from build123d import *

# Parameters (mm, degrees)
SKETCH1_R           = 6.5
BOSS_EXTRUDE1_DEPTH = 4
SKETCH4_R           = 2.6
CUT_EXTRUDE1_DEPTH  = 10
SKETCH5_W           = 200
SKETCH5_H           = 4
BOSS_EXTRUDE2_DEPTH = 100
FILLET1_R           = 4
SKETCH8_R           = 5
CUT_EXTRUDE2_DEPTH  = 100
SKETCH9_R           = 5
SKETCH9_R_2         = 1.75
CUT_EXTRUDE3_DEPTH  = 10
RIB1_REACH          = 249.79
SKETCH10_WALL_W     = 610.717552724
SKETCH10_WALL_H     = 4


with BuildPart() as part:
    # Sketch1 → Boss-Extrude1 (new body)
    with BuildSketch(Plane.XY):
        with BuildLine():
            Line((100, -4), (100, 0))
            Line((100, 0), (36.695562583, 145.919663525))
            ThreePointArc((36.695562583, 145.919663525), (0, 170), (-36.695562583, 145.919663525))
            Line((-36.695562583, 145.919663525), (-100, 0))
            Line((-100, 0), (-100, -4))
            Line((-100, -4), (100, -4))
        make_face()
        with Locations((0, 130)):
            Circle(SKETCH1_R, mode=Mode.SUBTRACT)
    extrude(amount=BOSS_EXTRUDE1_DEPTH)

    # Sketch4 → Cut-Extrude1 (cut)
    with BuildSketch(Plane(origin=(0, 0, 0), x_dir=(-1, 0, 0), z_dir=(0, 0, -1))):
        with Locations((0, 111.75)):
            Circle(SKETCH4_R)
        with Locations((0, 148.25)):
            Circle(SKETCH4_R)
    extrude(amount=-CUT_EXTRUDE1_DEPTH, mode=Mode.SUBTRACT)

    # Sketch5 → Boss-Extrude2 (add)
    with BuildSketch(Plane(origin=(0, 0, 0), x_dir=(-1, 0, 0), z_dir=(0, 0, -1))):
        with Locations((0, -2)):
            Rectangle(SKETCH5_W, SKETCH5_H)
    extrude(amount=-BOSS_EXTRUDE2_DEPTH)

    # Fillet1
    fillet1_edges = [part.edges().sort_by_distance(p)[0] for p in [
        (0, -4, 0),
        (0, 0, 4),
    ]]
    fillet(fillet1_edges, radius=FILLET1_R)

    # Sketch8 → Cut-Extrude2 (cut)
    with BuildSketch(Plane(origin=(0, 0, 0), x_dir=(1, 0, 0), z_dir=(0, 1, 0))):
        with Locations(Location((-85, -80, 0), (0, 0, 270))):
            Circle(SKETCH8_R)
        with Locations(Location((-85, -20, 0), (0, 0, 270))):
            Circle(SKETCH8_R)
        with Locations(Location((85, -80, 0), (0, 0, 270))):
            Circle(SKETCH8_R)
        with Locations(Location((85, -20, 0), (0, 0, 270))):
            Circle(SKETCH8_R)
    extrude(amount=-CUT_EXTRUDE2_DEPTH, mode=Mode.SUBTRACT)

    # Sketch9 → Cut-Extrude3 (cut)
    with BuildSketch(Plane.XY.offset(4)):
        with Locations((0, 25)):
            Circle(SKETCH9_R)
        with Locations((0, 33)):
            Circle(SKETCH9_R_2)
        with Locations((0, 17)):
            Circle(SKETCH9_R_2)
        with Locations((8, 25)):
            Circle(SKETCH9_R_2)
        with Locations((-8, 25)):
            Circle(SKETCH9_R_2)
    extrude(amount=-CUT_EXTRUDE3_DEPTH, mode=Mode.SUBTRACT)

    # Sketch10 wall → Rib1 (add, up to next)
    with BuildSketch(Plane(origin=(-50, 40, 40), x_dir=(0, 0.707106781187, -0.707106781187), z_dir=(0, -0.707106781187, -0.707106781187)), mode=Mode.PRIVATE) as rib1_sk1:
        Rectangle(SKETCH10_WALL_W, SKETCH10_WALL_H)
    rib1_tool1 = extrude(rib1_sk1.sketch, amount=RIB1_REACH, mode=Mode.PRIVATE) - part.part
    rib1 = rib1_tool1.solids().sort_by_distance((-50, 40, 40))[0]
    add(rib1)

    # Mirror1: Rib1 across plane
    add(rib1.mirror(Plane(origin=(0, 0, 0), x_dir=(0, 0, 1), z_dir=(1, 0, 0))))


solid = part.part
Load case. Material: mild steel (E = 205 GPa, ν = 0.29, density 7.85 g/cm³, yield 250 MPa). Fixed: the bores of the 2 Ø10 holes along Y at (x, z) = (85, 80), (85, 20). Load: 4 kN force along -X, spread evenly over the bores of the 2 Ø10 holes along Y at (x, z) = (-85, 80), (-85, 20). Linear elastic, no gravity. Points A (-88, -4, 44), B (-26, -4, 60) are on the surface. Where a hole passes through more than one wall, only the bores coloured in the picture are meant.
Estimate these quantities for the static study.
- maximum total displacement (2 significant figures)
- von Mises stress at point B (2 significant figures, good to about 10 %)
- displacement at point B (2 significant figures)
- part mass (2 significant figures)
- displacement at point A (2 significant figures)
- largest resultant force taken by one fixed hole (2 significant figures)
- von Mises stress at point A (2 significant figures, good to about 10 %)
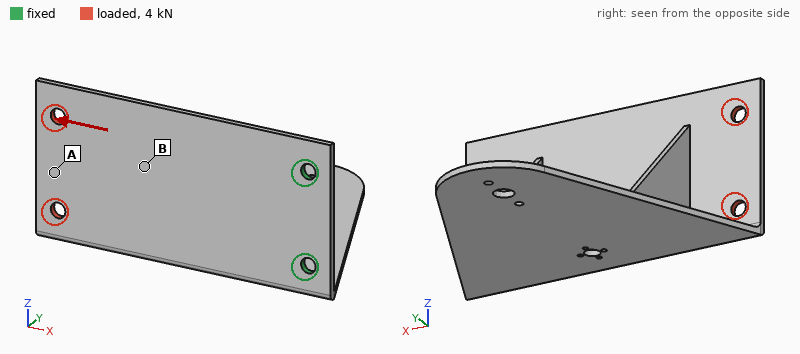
16 µm
9.7 MPa
7.3 µm
1.5 kg
13 µm
2.0 kN
3.4 MPa
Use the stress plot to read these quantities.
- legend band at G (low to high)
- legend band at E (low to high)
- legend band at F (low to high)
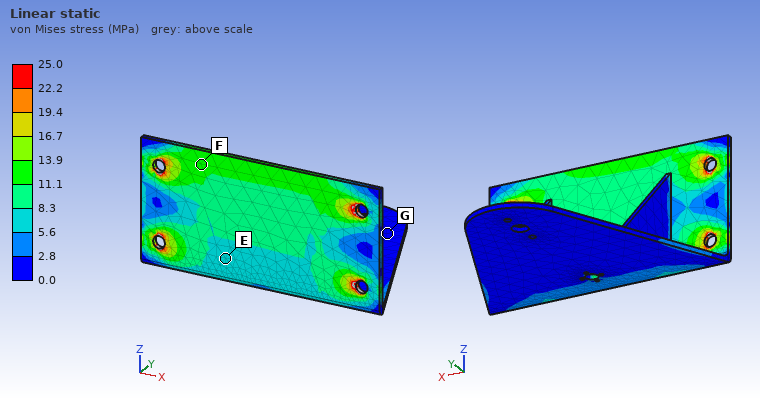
0.0 to 2.8 MPa
5.6 to 8.3 MPa
11.1 to 13.9 MPa
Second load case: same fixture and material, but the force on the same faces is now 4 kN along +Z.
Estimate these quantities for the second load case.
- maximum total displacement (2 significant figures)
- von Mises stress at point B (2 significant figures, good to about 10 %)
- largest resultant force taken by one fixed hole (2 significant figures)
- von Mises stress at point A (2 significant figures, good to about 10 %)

0.16 mm
24 MPa
11 kN
12 MPa
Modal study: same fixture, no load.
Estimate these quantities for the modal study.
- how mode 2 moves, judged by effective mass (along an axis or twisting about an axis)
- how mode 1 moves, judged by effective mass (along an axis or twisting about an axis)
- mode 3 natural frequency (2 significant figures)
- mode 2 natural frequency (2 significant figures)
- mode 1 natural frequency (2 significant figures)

along Z
along Y
520 Hz
200 Hz
110 Hz
